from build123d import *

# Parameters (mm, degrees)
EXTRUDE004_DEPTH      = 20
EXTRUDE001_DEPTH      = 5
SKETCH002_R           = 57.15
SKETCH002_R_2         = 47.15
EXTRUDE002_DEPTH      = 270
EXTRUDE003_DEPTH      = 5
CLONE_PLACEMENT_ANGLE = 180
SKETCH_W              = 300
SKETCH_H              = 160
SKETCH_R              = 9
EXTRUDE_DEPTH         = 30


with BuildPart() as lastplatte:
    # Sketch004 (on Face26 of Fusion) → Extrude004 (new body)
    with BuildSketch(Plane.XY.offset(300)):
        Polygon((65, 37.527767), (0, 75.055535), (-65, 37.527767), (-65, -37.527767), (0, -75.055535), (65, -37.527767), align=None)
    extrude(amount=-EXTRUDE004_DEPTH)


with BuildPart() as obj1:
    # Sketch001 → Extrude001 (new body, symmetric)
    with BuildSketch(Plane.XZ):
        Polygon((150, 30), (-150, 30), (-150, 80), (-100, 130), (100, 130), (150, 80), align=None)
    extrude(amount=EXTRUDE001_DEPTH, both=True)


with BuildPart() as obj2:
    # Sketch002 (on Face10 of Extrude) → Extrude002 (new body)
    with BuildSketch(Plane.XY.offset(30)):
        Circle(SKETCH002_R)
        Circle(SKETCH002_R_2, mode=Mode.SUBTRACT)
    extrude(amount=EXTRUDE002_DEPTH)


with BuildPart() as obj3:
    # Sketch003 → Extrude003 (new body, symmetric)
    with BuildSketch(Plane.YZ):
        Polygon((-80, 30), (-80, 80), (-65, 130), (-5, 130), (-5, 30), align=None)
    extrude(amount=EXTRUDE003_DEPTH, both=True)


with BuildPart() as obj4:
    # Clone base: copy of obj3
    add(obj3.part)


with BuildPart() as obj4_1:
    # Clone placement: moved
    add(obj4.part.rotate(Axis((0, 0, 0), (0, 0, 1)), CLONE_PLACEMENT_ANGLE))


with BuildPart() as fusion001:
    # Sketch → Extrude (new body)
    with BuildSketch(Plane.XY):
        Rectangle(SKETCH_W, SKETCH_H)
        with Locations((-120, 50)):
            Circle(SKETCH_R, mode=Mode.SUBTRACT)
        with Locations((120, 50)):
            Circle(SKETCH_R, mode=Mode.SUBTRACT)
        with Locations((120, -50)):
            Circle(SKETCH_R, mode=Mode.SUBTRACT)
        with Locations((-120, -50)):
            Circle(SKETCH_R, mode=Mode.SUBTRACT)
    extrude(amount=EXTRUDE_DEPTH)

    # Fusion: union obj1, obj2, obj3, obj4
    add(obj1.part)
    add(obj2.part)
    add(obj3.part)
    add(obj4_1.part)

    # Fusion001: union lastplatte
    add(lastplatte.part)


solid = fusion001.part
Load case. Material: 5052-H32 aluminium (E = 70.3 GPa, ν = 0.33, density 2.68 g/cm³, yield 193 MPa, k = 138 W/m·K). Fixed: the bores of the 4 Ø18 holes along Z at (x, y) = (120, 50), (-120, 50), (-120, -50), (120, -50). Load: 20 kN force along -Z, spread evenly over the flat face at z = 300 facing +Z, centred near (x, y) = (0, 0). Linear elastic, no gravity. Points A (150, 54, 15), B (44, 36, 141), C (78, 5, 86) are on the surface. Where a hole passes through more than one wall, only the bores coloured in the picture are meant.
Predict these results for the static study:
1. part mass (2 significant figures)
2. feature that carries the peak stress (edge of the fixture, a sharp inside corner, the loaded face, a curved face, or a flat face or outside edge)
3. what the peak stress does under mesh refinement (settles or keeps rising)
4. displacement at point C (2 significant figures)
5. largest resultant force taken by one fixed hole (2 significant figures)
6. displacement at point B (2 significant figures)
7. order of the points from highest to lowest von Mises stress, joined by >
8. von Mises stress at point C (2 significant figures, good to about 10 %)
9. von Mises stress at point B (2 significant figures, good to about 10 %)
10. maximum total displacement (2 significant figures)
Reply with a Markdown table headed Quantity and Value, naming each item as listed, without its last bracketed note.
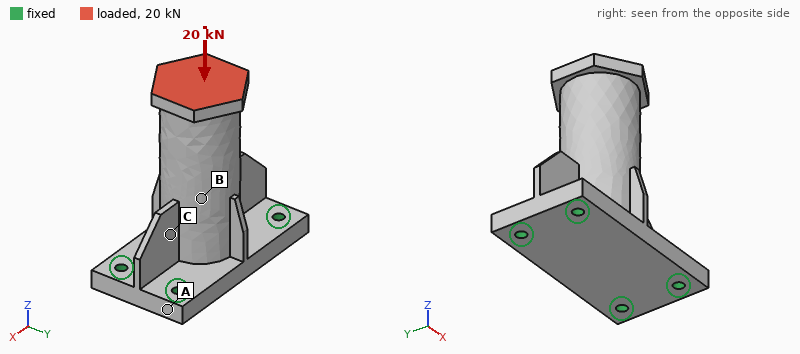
| Quantity | Value |
|---|---|
| part mass | 7.8 kg |
| feature that carries the peak stress | edge of the fixture |
| what the peak stress does under mesh refinement | keeps rising |
| displacement at point C | 16 µm |
| largest resultant force taken by one fixed hole | 5.3 kN |
| displacement at point B | 27 µm |
| order of the points from highest to lowest von Mises stress, joined by > | C > B > A |
| von Mises stress at point C | 8.0 MPa |
| von Mises stress at point B | 5.4 MPa |
| maximum total displacement | 46 µm |
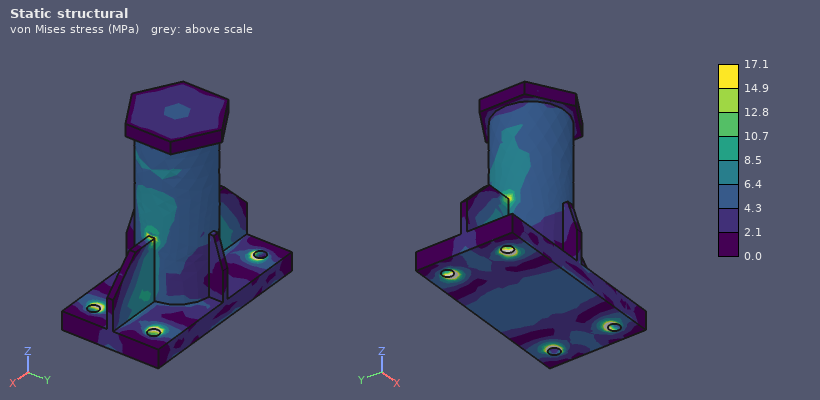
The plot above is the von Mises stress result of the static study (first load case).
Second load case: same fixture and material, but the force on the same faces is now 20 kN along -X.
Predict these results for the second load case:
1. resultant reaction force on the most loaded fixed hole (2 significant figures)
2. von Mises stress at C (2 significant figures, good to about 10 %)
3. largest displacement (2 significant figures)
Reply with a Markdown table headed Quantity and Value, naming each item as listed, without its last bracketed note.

| Quantity | Value |
|---|---|
| resultant reaction force on the most loaded fixed hole | 14 kN |
| von Mises stress at C | 31 MPa |
| largest displacement | 0.45 mm |
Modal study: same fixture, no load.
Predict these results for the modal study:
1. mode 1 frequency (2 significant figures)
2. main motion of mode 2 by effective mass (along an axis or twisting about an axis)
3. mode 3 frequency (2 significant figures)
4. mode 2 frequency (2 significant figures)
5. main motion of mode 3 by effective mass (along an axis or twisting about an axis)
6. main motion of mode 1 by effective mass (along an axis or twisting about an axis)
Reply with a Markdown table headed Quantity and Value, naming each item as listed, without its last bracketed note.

| Quantity | Value |
|---|---|
| mode 1 frequency | 500 Hz |
| main motion of mode 2 by effective mass | along X |
| mode 3 frequency | 2000 Hz |
| mode 2 frequency | 980 Hz |
| main motion of mode 3 by effective mass | along Z |
| main motion of mode 1 by effective mass | along Y |
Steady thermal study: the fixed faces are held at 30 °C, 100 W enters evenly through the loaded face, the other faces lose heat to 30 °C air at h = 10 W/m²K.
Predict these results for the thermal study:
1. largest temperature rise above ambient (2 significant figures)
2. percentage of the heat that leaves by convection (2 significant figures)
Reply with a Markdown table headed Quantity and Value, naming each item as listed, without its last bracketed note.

| Quantity | Value |
|---|---|
| largest temperature rise above ambient | 40 K |
| percentage of the heat that leaves by convection | 42 % |
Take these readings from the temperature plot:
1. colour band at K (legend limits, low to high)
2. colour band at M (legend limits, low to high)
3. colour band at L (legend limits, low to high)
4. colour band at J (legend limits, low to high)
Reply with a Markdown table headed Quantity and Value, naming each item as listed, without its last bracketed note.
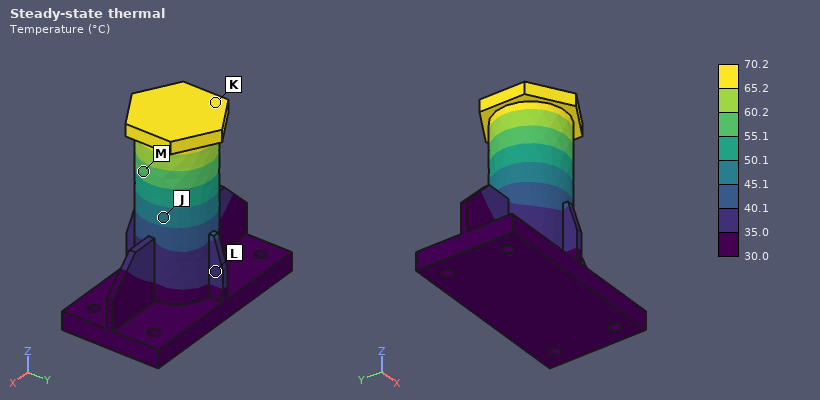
| Quantity | Value |
|---|---|
| colour band at K | 65.2 to 70.2 °C |
| colour band at M | 55.1 to 60.2 °C |
| colour band at L | 35.0 to 40.1 °C |
| colour band at J | 45.1 to 50.1 °C |
